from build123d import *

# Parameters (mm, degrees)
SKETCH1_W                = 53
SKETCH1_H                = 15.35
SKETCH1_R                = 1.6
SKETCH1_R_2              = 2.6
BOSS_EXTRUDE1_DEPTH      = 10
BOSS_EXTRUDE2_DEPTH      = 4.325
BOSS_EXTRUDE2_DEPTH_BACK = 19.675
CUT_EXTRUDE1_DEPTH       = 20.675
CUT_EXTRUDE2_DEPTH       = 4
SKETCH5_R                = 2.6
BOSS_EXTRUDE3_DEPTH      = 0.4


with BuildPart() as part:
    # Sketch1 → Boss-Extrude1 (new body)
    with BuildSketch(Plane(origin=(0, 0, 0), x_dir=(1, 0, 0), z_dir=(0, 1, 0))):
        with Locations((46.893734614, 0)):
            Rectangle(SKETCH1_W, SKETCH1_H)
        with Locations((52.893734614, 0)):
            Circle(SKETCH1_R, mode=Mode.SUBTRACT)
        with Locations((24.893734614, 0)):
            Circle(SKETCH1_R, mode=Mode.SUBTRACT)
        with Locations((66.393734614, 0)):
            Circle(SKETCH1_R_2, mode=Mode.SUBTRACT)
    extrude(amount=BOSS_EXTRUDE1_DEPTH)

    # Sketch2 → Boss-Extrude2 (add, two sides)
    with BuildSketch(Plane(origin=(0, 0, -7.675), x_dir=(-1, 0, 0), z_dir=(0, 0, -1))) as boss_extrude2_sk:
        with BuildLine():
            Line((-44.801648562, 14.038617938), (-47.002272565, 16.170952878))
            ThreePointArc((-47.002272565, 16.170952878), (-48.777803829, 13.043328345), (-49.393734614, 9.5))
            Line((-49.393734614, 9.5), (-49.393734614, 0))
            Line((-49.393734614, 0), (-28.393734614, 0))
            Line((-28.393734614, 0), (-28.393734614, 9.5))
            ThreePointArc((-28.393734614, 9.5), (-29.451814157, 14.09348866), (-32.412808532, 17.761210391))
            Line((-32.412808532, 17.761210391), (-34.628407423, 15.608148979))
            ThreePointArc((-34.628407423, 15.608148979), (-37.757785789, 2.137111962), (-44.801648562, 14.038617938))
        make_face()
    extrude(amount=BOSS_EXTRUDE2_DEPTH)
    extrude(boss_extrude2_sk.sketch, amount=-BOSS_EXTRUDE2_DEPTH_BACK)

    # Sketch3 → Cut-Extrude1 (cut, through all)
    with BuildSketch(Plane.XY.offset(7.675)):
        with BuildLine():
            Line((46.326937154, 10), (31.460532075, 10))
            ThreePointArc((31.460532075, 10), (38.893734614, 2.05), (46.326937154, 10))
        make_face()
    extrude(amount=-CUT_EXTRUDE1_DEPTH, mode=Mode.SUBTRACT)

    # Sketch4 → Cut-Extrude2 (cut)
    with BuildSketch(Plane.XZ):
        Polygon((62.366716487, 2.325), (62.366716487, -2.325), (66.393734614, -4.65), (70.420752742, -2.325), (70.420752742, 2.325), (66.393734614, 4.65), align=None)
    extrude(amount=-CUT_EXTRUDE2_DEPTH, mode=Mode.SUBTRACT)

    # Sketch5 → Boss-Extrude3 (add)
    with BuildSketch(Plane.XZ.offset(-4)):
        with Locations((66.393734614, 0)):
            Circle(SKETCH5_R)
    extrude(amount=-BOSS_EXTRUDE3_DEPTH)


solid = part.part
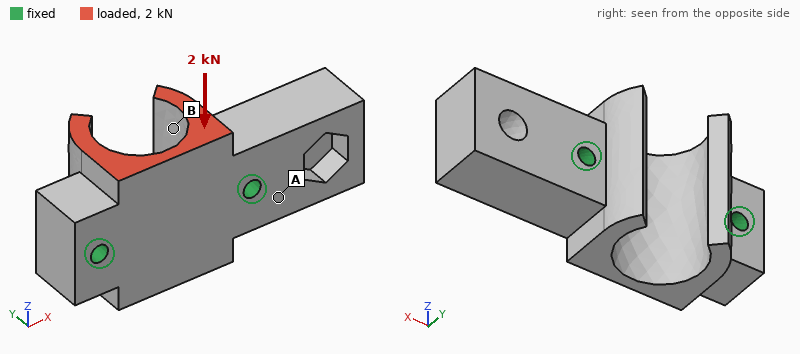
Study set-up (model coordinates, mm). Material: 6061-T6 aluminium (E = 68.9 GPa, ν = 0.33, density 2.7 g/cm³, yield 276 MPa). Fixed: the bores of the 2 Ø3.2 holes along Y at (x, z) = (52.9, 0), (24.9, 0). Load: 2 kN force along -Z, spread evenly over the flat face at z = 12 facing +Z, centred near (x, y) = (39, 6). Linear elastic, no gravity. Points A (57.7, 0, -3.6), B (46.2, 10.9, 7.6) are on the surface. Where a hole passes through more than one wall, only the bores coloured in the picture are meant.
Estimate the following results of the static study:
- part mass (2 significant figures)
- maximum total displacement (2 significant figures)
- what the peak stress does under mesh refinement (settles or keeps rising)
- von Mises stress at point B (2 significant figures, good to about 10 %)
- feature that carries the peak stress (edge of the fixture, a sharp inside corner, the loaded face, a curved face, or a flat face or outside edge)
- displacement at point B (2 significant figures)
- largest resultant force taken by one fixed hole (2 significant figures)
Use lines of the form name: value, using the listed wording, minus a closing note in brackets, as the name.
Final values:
part mass: 22 g
maximum total displacement: 12 µm
what the peak stress does under mesh refinement: keeps rising
von Mises stress at point B: 13 MPa
feature that carries the peak stress: edge of the fixture
displacement at point B: 5.3 µm
largest resultant force taken by one fixed hole: 1.0 kN
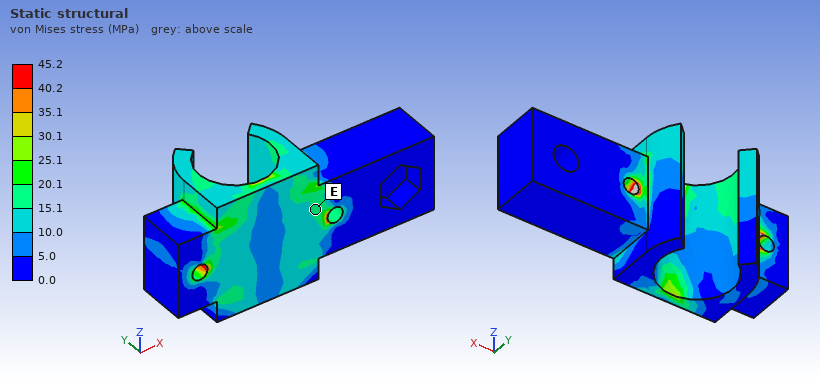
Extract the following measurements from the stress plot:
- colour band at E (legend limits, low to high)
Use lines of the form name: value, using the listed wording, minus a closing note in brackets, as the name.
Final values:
colour band at E: 15.1 to 20.1 MPa
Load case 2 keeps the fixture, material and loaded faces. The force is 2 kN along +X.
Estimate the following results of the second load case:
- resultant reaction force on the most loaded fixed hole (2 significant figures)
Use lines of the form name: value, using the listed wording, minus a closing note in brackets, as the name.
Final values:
resultant reaction force on the most loaded fixed hole: 1.3 kN
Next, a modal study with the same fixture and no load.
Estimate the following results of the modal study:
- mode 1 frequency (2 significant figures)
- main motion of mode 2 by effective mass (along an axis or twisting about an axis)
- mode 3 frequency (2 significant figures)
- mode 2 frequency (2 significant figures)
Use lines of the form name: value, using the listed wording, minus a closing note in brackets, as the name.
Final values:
mode 1 frequency: 15 kHz
main motion of mode 2 by effective mass: along Y
mode 3 frequency: 23 kHz
mode 2 frequency: 16 kHz
